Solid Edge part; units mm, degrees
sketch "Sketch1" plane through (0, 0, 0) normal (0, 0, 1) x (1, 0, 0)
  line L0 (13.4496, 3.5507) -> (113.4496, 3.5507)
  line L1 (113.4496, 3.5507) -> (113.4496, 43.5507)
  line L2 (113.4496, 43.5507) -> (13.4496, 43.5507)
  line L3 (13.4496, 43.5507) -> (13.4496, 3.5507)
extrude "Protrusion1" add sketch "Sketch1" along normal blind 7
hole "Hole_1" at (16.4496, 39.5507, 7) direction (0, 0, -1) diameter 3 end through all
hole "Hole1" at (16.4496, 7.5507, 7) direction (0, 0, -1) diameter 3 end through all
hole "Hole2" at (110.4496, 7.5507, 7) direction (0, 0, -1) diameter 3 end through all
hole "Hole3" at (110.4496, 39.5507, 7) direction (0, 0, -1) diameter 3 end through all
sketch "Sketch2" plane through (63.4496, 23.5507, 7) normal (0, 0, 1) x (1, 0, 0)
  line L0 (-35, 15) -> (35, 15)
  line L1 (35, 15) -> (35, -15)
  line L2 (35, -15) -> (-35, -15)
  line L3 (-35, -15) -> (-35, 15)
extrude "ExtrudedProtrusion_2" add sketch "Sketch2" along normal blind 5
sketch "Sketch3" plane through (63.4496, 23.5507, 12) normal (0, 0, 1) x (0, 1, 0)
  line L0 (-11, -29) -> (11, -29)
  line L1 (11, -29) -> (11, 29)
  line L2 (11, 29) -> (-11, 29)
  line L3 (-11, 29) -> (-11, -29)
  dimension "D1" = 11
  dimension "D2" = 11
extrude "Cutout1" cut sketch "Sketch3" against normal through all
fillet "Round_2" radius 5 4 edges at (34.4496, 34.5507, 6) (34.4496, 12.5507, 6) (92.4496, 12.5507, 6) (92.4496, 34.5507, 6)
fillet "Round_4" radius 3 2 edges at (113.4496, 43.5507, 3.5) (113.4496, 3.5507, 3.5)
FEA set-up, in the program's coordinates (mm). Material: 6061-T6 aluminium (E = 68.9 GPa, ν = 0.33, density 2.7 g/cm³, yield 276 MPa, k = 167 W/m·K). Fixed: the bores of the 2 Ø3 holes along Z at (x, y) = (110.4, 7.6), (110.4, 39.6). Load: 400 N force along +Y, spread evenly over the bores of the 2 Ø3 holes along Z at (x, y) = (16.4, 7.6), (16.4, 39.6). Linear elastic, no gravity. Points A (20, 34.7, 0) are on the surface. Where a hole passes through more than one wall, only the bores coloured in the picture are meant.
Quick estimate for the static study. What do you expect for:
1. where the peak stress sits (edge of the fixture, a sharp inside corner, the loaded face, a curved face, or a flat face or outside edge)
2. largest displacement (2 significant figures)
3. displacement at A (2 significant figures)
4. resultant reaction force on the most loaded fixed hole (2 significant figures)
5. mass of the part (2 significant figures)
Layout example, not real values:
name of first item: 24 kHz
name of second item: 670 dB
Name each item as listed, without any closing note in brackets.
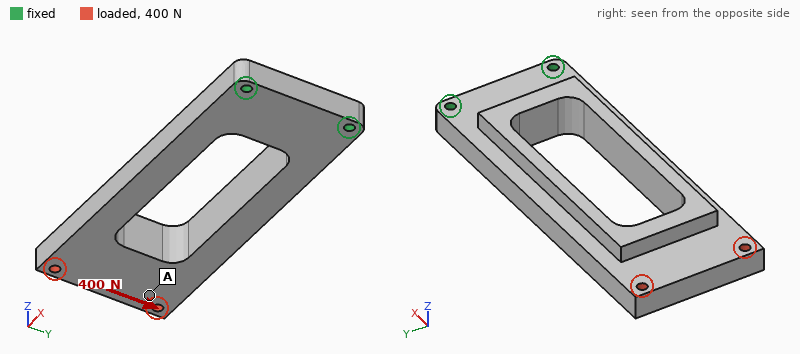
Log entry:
where the peak stress sits: a curved face
largest displacement: 0.18 mm
displacement at A: 0.18 mm
resultant reaction force on the most loaded fixed hole: 1.2 kN
mass of the part: 63 g
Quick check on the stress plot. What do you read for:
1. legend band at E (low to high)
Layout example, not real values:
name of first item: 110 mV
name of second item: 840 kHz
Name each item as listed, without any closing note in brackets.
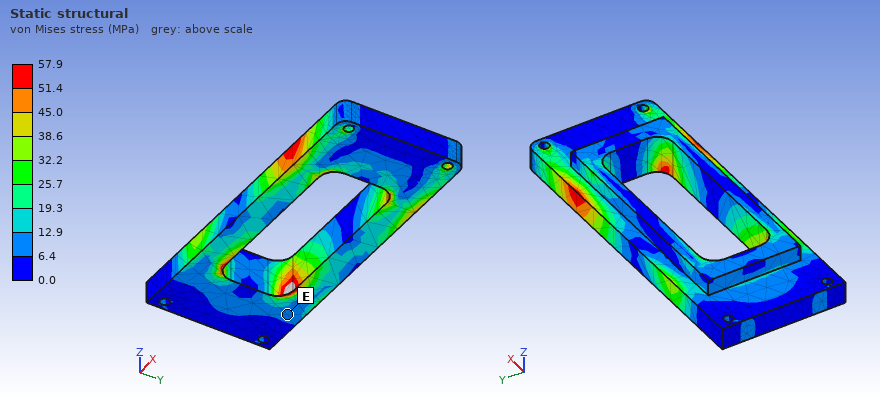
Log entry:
legend band at E: 6.4 to 12.9 MPa
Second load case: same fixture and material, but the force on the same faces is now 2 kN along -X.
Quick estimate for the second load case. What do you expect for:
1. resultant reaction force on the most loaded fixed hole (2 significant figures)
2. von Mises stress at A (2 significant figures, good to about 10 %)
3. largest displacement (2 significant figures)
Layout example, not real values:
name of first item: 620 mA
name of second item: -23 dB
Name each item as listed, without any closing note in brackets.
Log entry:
resultant reaction force on the most loaded fixed hole: 1.0 kN
von Mises stress at A: 8.6 MPa
largest displacement: 86 µm
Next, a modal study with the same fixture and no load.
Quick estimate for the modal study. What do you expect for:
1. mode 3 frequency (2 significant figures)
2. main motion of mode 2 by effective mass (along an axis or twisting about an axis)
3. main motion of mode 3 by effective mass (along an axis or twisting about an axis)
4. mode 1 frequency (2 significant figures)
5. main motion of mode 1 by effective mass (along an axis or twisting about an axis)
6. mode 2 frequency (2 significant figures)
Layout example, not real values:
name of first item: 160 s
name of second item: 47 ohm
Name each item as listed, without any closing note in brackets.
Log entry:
mode 3 frequency: 2300 Hz
main motion of mode 2 by effective mass: along Y
main motion of mode 3 by effective mass: twisting about X
mode 1 frequency: 610 Hz
main motion of mode 1 by effective mass: along Z
mode 2 frequency: 1500 Hz
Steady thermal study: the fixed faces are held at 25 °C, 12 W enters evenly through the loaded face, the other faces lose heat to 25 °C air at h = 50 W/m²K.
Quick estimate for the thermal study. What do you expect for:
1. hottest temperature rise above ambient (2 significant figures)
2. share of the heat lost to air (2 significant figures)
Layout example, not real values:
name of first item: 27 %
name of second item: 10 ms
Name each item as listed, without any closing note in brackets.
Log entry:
hottest temperature rise above ambient: 26 K
share of the heat lost to air: 47 %
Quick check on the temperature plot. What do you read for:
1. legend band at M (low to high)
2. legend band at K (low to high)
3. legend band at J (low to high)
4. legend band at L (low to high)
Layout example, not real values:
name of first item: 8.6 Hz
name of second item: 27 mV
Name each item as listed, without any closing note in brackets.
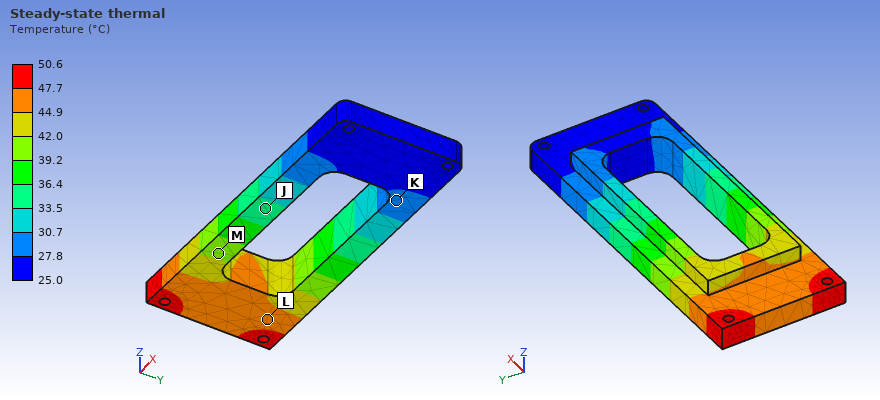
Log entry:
legend band at M: 39.2 to 42.0 °C
legend band at K: 27.8 to 30.7 °C
legend band at J: 33.5 to 36.4 °C
legend band at L: 44.9 to 47.7 °C
